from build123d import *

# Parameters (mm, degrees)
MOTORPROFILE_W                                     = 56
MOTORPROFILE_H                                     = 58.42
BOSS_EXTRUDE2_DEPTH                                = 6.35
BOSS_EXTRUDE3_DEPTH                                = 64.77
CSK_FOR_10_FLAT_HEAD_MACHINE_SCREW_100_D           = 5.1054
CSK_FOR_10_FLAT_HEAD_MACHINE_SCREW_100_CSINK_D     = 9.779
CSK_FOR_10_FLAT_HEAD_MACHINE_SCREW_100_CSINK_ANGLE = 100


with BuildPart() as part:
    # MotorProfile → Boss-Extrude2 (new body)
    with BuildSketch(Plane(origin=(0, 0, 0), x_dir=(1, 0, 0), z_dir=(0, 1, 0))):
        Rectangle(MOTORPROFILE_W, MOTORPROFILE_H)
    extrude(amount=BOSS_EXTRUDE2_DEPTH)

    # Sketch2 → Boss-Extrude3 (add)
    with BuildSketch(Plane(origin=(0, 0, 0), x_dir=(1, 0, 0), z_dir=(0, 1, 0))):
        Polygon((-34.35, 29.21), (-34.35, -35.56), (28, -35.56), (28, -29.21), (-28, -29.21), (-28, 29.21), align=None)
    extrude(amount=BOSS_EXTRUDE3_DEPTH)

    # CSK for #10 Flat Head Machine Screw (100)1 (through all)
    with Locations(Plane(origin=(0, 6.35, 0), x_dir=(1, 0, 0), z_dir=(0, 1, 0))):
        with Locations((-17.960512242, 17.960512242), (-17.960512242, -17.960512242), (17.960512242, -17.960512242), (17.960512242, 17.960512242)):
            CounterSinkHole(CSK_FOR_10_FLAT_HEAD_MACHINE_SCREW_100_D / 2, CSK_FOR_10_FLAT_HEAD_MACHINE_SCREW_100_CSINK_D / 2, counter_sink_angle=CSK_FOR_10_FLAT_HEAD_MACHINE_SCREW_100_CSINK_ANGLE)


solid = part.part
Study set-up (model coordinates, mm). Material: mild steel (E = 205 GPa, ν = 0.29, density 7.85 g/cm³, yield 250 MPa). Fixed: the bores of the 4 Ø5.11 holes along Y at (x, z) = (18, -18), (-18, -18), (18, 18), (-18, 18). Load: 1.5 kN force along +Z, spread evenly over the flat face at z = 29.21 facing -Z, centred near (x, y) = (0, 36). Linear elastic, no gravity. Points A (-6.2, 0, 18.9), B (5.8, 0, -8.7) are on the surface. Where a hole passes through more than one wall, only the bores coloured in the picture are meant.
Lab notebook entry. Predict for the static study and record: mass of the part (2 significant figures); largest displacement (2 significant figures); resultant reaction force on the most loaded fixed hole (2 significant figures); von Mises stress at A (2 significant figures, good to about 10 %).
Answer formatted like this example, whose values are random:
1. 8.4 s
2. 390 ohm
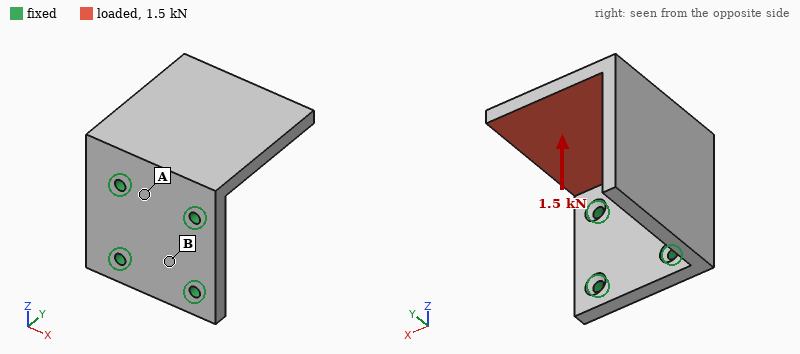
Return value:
1. 550 g
2. 0.12 mm
3. 1.2 kN
4. 22 MPa
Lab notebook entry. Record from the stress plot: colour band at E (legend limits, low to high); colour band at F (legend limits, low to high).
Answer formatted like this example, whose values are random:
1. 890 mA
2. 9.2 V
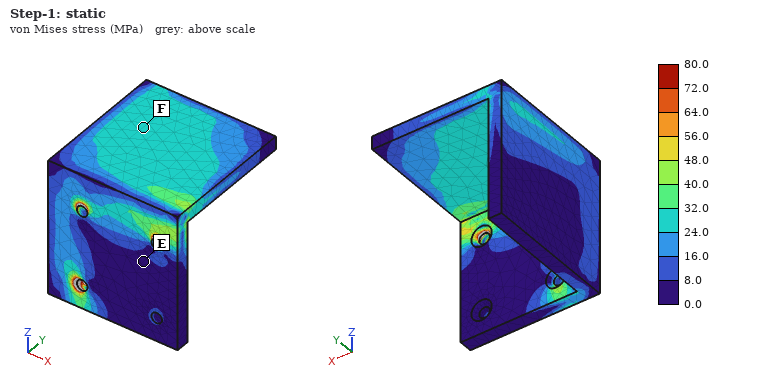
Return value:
1. 0.0 to 8.0 MPa
2. 24.0 to 32.0 MPa
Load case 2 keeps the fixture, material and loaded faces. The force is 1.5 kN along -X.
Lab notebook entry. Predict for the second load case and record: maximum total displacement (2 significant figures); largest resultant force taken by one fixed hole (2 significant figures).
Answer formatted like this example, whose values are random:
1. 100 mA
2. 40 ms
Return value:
1. 36 µm
2. 1.6 kN
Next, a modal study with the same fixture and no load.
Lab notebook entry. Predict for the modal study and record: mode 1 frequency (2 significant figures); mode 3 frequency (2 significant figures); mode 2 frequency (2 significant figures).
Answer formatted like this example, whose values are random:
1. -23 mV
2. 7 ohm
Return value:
1. 1600 Hz
2. 3000 Hz
3. 2100 Hz
